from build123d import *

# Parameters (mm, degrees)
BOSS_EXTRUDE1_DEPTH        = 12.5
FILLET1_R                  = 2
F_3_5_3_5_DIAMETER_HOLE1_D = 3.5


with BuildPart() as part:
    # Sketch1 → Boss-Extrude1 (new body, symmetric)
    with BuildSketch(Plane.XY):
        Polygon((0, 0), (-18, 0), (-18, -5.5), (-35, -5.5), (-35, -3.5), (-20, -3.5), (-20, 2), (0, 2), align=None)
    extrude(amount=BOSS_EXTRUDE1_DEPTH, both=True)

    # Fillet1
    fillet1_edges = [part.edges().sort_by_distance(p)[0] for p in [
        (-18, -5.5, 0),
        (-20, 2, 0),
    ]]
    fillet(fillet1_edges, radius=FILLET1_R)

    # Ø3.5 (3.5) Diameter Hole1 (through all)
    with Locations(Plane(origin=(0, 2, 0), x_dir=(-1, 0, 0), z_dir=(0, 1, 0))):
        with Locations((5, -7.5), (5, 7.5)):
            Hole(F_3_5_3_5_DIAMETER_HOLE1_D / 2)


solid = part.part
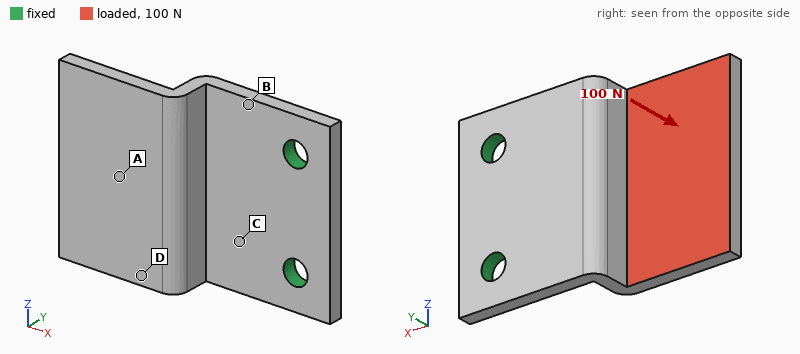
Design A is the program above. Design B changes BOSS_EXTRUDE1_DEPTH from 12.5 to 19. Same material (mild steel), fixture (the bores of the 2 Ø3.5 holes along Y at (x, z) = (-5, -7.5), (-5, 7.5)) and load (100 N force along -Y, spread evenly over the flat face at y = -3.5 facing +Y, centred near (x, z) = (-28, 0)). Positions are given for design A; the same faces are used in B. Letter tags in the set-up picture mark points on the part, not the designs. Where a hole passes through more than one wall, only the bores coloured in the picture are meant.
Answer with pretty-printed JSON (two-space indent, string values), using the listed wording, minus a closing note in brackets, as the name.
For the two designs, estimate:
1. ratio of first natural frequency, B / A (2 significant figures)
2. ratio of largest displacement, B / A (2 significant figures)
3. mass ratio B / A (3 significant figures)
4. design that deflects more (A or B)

{
  "ratio of first natural frequency, B / A": "0.95",
  "ratio of largest displacement, B / A": "0.71",
  "mass ratio B / A": "1.53",
  "design that deflects more": "A"
}
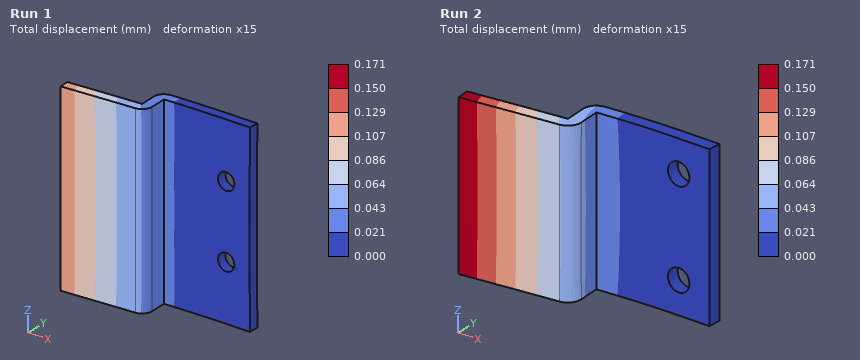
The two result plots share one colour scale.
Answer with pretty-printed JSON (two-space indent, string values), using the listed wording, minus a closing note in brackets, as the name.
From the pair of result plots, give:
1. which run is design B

{
  "which run is design B": "Run 1"
}
